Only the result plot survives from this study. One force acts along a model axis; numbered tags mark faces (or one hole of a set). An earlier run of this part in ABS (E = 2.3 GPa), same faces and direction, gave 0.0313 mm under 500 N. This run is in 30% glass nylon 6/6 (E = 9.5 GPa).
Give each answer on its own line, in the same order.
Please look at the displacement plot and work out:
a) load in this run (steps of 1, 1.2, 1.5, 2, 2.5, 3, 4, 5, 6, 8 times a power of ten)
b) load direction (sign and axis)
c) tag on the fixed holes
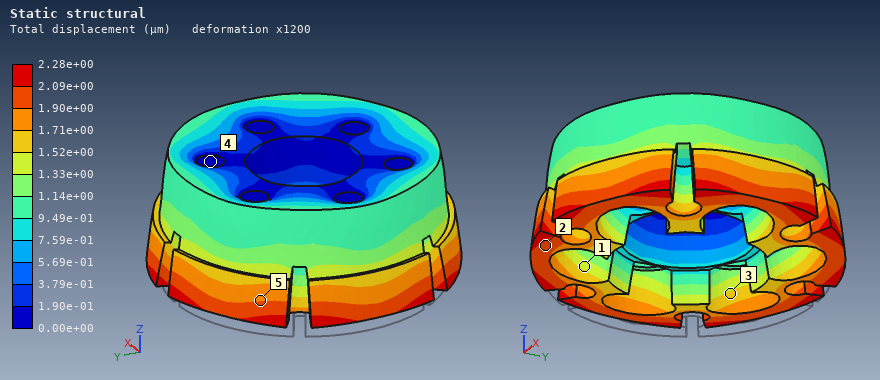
150 N
+Z
4
